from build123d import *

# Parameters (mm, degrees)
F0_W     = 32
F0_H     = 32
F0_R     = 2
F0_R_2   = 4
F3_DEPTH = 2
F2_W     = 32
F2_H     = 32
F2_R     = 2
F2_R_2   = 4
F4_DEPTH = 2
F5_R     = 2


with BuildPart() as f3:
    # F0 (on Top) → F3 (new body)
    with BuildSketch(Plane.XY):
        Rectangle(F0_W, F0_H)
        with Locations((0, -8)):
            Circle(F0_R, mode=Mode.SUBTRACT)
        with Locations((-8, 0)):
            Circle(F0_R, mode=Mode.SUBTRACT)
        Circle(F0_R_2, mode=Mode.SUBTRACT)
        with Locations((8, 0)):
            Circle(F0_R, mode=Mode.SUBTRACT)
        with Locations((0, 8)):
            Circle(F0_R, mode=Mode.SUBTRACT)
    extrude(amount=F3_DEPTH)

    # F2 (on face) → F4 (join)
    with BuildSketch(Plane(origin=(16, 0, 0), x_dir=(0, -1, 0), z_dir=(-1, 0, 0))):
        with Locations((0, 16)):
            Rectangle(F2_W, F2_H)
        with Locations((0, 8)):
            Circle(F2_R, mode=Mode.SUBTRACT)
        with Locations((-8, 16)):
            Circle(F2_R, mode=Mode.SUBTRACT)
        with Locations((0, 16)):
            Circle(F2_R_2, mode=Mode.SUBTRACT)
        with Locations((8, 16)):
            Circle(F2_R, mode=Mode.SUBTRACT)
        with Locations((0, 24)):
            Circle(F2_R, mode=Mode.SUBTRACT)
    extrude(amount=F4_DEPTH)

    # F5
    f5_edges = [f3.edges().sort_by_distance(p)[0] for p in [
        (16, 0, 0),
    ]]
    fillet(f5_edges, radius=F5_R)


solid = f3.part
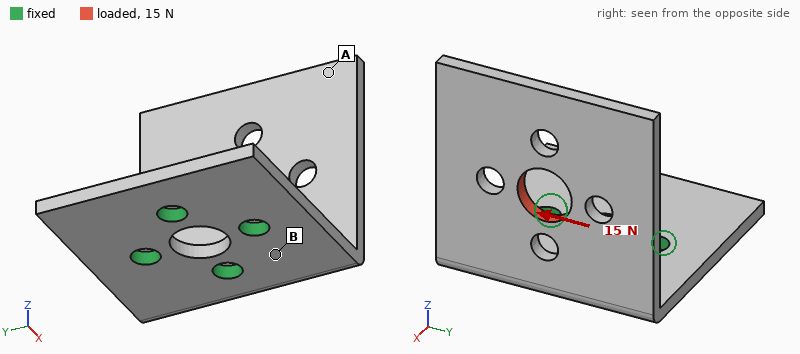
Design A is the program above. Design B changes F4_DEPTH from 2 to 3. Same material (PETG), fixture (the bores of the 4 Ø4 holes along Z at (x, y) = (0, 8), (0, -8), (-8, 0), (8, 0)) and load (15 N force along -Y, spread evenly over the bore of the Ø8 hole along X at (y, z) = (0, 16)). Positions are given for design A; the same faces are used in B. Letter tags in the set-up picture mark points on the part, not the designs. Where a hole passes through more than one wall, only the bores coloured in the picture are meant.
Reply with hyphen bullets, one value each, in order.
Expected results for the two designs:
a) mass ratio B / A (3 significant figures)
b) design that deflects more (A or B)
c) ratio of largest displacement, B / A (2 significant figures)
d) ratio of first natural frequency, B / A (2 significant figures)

- 1.24
- A
- 0.69
- 1.1
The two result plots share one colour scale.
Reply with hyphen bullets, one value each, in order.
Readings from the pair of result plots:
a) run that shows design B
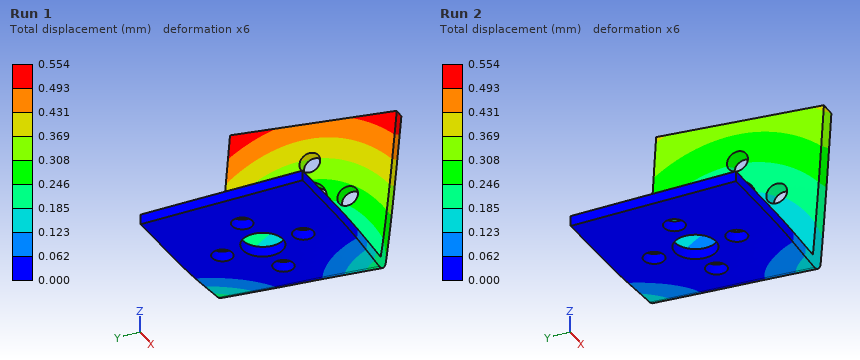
- Run 2
